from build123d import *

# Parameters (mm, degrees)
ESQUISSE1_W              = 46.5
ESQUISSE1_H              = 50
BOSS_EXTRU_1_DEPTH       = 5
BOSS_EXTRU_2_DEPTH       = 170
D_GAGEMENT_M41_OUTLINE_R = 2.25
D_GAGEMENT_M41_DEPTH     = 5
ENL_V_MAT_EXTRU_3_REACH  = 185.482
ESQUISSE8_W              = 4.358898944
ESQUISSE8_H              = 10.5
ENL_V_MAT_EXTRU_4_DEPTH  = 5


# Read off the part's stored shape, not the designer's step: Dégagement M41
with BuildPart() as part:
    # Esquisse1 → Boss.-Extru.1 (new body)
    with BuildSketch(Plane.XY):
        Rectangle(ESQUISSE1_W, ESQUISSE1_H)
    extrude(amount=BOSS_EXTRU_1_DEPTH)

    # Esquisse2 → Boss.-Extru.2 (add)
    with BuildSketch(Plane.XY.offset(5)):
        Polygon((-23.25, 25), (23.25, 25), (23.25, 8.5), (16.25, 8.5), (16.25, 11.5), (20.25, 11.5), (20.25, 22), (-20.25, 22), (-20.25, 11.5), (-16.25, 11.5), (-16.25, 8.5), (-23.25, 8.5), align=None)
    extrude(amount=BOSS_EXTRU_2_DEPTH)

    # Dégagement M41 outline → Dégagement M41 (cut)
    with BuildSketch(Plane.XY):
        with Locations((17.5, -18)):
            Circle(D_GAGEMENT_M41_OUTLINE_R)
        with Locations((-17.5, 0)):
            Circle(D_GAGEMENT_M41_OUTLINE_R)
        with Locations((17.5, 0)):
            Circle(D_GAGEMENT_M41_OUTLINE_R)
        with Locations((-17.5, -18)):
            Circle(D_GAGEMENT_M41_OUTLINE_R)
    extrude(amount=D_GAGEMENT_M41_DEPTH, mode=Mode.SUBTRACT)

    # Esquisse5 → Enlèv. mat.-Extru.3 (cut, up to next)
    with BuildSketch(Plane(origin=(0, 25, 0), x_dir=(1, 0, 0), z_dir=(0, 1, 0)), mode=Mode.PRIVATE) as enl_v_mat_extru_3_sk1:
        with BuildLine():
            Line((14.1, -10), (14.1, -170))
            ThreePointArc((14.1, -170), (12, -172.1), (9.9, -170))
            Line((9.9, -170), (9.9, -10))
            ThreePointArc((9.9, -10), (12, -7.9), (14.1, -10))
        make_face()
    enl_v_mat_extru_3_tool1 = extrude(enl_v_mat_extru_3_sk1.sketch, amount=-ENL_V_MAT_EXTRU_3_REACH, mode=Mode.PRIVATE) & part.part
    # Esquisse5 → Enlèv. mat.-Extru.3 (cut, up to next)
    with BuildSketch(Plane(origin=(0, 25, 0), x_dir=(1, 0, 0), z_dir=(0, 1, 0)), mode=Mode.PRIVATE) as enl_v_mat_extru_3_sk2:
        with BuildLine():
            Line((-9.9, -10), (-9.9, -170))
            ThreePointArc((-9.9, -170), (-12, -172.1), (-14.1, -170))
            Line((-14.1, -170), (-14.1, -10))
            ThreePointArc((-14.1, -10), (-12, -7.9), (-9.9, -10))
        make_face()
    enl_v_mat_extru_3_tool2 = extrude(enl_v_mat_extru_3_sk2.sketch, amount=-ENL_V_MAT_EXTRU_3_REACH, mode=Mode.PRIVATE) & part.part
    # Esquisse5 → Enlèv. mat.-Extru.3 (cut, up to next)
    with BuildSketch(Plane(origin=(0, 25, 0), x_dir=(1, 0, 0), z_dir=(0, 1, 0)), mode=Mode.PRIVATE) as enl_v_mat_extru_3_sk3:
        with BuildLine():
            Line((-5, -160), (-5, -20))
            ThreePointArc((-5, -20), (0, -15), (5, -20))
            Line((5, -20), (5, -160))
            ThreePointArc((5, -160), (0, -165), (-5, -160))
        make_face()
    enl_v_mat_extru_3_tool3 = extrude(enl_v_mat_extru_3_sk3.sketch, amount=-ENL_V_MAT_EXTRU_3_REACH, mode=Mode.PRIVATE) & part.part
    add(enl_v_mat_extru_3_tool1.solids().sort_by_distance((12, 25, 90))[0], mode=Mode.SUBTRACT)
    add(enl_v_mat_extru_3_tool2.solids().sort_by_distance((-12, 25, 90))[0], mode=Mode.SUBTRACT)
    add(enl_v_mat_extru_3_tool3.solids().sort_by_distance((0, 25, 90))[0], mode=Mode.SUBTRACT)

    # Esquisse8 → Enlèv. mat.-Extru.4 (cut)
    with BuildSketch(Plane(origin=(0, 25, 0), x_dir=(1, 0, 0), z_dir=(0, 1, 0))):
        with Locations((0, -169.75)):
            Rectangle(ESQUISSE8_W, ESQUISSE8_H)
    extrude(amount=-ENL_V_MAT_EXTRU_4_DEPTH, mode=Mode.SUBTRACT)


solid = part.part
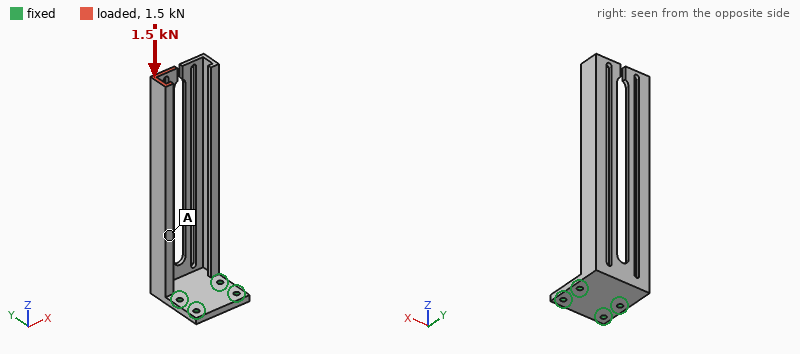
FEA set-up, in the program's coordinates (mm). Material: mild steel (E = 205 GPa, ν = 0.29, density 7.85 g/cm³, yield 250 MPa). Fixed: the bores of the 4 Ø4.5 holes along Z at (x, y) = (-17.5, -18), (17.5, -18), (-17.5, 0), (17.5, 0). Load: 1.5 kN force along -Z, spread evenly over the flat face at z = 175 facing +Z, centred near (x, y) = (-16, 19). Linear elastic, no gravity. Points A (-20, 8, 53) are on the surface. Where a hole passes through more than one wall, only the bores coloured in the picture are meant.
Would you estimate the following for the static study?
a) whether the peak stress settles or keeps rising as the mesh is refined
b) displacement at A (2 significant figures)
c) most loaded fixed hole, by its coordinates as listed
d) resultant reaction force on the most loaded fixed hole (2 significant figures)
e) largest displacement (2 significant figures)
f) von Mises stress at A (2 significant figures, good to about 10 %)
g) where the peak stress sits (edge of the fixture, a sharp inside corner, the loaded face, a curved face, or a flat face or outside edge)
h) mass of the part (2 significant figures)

keeps rising
0.20 mm
(-17.5, 0)
1.7 kN
0.70 mm
13 MPa
edge of the fixture
350 g
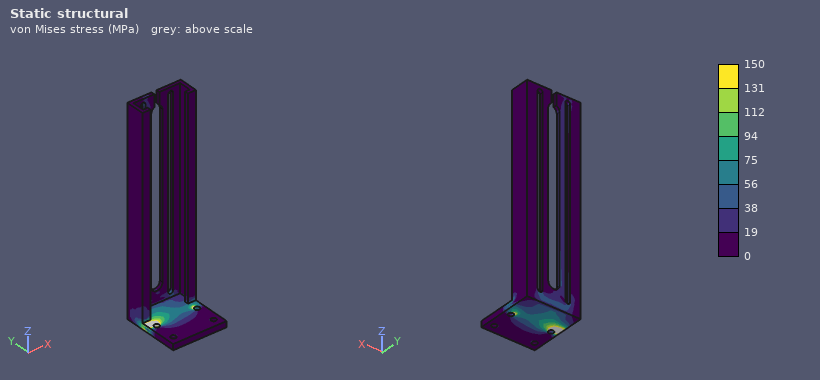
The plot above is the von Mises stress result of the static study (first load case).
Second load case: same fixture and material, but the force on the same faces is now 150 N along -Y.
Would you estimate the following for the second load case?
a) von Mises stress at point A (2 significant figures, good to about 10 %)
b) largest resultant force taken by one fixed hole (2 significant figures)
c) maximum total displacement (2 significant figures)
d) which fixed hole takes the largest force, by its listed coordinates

70 MPa
300 N
1.8 mm
(-17.5, 0)
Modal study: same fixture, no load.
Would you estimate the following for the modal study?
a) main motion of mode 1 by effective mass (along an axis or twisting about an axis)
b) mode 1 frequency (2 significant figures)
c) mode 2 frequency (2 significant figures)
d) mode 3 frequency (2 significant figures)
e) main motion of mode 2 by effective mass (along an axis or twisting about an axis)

along X
200 Hz
220 Hz
240 Hz
along Y
